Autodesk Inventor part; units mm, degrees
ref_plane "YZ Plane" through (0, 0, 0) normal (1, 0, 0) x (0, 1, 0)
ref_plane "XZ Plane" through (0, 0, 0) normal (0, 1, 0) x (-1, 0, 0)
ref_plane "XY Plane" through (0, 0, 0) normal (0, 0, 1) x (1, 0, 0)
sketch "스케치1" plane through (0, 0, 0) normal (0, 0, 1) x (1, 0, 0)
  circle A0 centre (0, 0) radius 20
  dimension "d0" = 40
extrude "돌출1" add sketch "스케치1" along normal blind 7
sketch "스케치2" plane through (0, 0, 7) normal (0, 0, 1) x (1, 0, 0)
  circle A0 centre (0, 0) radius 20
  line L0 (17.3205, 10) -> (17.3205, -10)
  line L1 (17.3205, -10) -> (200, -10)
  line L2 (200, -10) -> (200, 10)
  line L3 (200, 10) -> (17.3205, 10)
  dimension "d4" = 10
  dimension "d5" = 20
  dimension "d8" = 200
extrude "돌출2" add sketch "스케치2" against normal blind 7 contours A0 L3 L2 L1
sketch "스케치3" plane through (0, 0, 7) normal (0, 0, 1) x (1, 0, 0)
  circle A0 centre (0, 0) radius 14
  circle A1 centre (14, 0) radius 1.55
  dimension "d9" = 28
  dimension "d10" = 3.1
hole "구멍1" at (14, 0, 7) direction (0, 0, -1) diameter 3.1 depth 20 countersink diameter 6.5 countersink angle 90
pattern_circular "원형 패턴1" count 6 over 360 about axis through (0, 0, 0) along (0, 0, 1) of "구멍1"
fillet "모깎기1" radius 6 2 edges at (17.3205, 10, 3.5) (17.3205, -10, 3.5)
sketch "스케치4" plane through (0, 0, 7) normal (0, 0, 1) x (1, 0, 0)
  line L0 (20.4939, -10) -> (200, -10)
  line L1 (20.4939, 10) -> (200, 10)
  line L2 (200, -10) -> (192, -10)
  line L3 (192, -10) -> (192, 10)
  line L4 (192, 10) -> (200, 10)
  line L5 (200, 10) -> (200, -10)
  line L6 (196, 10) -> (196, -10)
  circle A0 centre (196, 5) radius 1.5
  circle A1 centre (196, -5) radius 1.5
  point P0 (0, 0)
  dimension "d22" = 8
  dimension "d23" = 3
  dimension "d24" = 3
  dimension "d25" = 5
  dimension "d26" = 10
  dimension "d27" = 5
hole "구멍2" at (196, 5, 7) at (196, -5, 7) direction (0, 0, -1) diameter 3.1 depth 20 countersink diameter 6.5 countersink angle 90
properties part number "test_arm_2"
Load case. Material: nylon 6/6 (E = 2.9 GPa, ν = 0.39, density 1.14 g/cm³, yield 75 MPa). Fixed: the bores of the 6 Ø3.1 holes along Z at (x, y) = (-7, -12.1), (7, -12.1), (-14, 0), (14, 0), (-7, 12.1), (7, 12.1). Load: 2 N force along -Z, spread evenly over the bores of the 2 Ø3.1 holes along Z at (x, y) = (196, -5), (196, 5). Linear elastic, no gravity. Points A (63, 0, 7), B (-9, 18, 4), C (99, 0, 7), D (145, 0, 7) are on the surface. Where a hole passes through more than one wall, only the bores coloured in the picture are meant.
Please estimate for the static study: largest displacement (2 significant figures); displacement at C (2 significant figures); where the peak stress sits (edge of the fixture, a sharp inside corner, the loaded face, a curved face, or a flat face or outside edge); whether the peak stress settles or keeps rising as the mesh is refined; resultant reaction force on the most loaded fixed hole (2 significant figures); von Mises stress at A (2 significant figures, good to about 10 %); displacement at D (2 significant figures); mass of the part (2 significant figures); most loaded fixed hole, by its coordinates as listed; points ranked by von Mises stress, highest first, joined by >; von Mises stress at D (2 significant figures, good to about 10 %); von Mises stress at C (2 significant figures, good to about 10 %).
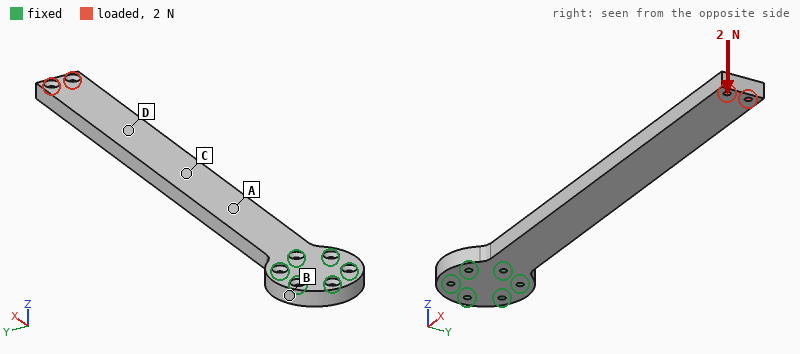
2.5 mm
0.69 mm
edge of the fixture
keeps rising
21 N
1.6 MPa
1.5 mm
38 g
(14, 0)
A > C > D > B
0.63 MPa
1.2 MPa
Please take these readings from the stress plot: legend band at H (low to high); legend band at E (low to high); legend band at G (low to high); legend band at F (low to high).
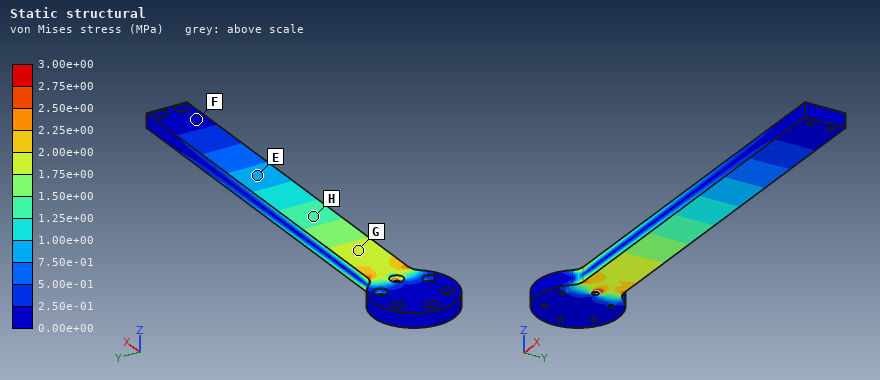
1.25e+00 to 1.50e+00 MPa
7.50e-01 to 1.00e+00 MPa
1.75e+00 to 2.00e+00 MPa
0.00e+00 to 2.50e-01 MPa
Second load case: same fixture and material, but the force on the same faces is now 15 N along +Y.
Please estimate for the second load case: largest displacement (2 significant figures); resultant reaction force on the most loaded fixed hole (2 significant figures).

2.4 mm
97 N
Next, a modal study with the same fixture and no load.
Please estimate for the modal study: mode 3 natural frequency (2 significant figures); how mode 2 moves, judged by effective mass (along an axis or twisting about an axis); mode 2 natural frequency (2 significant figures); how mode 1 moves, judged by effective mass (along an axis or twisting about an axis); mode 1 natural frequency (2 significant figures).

320 Hz
along Y
150 Hz
along Z
52 Hz
